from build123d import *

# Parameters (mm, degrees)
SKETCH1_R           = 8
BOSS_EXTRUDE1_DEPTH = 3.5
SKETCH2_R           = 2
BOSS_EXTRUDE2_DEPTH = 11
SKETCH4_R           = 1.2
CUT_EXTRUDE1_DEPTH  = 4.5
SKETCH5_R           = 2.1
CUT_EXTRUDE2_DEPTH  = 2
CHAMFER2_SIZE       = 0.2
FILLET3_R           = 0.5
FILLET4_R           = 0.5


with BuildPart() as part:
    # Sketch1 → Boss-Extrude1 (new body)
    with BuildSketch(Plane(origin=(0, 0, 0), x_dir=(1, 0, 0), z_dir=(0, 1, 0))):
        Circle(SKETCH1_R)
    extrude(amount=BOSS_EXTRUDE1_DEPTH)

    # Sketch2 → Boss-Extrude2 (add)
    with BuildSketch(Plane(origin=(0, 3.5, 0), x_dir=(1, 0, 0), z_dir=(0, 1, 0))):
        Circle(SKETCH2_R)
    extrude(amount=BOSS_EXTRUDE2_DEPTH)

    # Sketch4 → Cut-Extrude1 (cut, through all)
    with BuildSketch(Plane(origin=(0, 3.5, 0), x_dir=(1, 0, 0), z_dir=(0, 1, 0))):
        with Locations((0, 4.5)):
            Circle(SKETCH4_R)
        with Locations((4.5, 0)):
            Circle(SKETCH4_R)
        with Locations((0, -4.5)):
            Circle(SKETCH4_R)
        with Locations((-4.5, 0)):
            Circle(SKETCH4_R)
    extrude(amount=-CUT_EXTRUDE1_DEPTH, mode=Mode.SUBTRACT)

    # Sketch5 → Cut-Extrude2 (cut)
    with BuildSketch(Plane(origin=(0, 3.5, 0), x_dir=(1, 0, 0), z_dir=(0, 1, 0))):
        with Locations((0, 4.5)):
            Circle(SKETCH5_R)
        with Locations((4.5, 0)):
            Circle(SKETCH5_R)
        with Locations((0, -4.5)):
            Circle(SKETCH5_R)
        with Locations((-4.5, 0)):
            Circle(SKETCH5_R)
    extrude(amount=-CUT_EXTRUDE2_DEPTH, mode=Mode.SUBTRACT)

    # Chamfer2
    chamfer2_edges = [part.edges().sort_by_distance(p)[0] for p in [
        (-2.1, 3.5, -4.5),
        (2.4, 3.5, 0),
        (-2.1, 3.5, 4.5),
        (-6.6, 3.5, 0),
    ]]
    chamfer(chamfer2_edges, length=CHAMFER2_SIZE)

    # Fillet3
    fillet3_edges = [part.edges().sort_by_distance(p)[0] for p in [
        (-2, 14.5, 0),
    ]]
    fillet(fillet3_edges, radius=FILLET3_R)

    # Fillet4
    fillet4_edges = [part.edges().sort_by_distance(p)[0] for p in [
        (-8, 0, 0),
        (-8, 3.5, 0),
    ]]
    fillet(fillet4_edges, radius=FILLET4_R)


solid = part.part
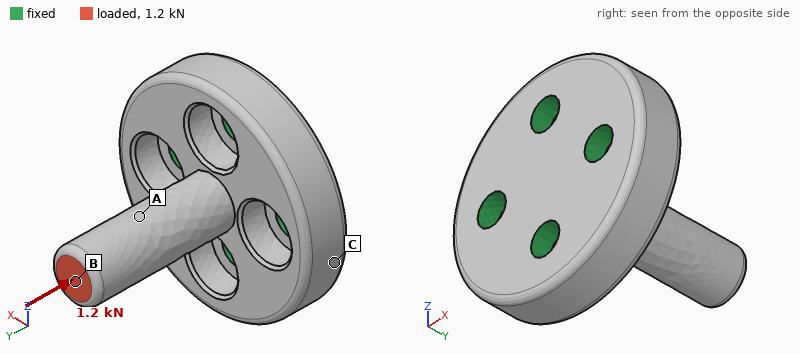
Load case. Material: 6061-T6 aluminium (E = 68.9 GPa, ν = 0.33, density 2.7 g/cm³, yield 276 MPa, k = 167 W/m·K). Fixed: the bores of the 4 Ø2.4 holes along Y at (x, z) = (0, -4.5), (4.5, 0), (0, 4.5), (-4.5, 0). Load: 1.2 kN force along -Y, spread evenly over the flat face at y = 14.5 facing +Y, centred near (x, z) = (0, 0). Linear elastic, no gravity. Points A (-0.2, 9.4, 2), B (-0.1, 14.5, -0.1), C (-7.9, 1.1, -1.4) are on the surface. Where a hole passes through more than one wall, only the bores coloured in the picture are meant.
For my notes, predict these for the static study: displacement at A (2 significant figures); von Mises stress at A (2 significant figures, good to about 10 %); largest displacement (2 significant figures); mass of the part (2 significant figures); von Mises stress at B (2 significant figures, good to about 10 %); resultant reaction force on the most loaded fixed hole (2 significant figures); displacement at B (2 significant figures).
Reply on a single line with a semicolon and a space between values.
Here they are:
13 µm; 96 MPa; 22 µm; 1.9 g; 85 MPa; 330 N; 22 µm
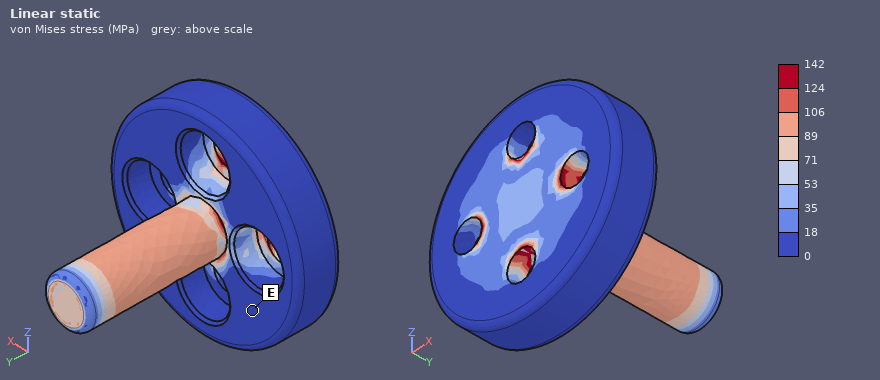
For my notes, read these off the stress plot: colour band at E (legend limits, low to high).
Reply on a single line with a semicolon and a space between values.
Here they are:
0 to 18 MPa
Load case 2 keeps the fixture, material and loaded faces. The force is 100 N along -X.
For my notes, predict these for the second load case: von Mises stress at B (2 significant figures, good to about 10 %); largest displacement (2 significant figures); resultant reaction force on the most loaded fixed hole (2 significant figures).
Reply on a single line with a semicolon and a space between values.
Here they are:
25 MPa; 75 µm; 160 N
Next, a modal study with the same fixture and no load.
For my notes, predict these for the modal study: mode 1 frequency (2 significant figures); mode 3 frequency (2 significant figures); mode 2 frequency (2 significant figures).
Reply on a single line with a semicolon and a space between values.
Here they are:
18 kHz; 66 kHz; 18 kHz
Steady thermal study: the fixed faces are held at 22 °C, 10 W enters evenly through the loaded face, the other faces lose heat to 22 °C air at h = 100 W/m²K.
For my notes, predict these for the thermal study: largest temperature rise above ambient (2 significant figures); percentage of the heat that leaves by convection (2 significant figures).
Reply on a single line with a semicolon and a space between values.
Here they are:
62 K; 5.4 %
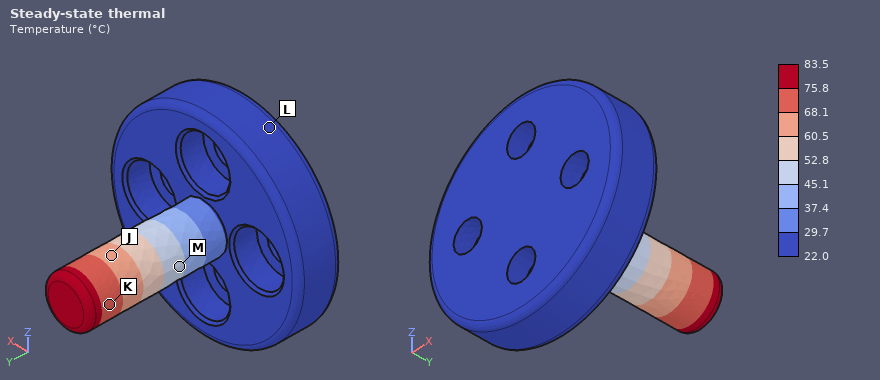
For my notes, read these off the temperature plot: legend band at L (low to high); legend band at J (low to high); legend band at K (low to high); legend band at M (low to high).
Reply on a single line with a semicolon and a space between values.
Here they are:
22.0 to 29.7 °C; 60.5 to 68.1 °C; 68.1 to 75.8 °C; 45.1 to 52.8 °C
